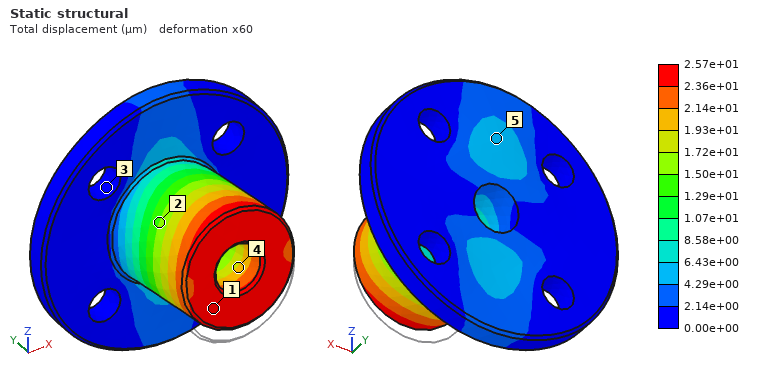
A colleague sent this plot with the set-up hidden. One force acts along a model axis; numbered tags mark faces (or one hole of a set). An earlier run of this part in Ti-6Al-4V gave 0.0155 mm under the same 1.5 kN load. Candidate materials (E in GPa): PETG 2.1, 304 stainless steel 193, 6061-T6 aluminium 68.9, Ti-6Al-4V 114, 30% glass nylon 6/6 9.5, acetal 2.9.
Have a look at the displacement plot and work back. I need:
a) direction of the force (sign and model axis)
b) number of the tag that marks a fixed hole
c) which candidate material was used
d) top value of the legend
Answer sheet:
+Z
3
6061-T6 aluminium
2.57e+01 µm
